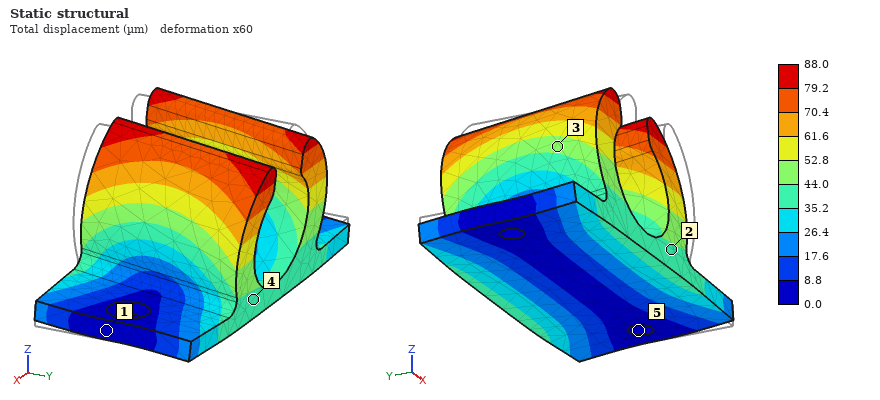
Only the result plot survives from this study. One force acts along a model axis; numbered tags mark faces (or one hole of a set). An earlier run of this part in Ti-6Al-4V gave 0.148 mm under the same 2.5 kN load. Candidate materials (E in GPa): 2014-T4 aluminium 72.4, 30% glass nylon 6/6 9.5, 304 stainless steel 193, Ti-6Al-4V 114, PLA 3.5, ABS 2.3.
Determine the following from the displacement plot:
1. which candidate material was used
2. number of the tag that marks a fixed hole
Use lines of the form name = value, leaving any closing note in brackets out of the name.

which candidate material was used = 304 stainless steel
number of the tag that marks a fixed hole = 5
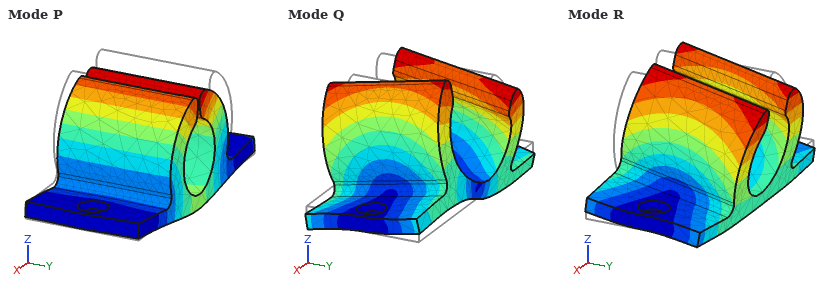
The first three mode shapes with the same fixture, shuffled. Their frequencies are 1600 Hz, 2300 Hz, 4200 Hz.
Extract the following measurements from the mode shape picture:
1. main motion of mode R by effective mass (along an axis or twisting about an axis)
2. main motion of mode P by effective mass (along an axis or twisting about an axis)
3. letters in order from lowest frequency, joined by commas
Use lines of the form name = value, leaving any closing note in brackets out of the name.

main motion of mode R by effective mass = along Y
main motion of mode P by effective mass = along Z
letters in order from lowest frequency, joined by commas = R, P, Q
